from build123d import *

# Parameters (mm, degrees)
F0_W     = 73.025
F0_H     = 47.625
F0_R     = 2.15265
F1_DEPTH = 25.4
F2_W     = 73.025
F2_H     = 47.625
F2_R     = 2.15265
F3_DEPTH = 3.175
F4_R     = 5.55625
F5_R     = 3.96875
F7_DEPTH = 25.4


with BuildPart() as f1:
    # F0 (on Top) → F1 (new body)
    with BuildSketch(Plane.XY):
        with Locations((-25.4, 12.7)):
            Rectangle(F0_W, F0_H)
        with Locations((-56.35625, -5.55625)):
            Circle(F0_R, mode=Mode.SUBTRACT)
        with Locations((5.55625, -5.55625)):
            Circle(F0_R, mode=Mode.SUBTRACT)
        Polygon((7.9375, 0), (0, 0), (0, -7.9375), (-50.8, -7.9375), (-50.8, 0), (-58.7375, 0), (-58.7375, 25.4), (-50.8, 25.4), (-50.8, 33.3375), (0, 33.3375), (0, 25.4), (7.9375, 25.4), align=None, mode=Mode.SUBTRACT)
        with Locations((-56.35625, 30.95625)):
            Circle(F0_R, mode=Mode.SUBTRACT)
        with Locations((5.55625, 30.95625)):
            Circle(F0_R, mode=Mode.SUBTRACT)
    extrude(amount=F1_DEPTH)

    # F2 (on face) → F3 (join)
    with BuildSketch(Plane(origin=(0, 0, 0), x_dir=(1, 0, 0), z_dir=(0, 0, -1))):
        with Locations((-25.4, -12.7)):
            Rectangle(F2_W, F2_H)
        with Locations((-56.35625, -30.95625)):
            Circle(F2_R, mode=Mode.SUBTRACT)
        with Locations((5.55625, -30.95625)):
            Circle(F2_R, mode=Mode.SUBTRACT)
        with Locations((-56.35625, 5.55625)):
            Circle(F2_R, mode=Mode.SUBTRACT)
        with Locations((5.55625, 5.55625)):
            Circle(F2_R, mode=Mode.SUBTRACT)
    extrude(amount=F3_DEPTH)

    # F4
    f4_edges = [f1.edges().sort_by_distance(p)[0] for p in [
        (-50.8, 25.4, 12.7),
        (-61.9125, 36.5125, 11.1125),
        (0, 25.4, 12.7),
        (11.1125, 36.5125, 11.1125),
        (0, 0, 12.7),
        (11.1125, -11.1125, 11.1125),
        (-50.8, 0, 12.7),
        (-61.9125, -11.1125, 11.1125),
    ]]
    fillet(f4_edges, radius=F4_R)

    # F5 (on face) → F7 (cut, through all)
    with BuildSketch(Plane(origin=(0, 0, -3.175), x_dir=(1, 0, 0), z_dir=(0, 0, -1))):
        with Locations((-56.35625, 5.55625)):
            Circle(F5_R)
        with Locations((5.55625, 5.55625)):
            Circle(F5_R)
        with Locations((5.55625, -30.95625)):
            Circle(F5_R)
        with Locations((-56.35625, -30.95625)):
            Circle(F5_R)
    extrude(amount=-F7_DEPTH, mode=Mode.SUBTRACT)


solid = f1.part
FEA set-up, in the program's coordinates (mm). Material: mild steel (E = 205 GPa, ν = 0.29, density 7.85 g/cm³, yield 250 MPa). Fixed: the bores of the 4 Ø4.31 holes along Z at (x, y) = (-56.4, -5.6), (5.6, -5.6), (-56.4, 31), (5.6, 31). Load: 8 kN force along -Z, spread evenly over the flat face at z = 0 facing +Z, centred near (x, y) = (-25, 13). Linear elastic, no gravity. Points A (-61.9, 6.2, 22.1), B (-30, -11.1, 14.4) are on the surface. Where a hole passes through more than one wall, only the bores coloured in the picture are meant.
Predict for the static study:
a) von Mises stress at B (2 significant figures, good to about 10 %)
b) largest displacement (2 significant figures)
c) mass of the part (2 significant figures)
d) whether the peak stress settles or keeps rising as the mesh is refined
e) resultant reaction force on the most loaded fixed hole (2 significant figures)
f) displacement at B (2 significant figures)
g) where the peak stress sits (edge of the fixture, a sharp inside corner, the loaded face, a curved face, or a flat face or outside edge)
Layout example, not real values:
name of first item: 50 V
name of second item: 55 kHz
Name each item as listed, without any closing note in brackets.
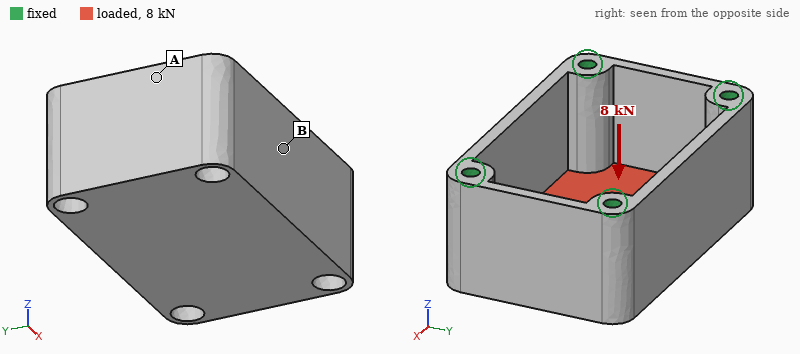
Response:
von Mises stress at B: 40 MPa
largest displacement: 85 µm
mass of the part: 230 g
whether the peak stress settles or keeps rising as the mesh is refined: keeps rising
resultant reaction force on the most loaded fixed hole: 2.1 kN
displacement at B: 26 µm
where the peak stress sits: edge of the fixture
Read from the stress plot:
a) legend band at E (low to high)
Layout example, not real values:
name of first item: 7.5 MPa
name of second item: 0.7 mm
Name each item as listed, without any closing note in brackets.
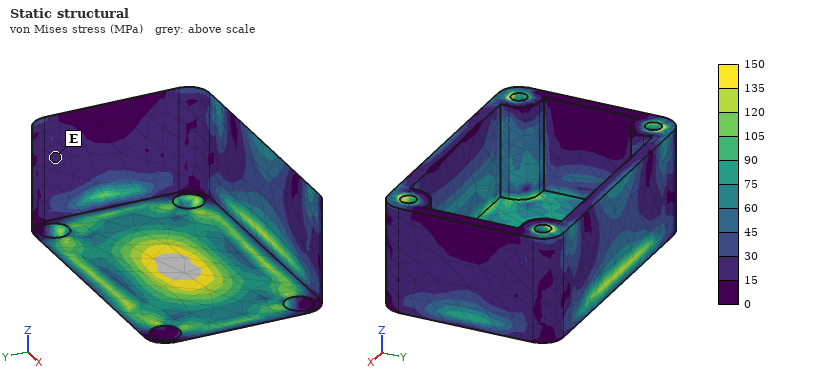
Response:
legend band at E: 15 to 30 MPa
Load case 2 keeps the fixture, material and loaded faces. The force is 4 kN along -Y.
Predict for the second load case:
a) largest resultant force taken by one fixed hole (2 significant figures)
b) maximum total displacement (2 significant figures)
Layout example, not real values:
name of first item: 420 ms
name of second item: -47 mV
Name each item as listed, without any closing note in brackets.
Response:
largest resultant force taken by one fixed hole: 1.6 kN
maximum total displacement: 15 µm
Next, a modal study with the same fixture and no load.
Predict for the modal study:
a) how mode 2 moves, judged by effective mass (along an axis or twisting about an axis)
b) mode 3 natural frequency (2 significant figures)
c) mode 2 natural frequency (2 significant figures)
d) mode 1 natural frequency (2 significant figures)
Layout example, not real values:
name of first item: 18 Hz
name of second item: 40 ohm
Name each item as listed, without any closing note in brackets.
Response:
how mode 2 moves, judged by effective mass: along Y
mode 3 natural frequency: 8600 Hz
mode 2 natural frequency: 6700 Hz
mode 1 natural frequency: 6300 Hz
